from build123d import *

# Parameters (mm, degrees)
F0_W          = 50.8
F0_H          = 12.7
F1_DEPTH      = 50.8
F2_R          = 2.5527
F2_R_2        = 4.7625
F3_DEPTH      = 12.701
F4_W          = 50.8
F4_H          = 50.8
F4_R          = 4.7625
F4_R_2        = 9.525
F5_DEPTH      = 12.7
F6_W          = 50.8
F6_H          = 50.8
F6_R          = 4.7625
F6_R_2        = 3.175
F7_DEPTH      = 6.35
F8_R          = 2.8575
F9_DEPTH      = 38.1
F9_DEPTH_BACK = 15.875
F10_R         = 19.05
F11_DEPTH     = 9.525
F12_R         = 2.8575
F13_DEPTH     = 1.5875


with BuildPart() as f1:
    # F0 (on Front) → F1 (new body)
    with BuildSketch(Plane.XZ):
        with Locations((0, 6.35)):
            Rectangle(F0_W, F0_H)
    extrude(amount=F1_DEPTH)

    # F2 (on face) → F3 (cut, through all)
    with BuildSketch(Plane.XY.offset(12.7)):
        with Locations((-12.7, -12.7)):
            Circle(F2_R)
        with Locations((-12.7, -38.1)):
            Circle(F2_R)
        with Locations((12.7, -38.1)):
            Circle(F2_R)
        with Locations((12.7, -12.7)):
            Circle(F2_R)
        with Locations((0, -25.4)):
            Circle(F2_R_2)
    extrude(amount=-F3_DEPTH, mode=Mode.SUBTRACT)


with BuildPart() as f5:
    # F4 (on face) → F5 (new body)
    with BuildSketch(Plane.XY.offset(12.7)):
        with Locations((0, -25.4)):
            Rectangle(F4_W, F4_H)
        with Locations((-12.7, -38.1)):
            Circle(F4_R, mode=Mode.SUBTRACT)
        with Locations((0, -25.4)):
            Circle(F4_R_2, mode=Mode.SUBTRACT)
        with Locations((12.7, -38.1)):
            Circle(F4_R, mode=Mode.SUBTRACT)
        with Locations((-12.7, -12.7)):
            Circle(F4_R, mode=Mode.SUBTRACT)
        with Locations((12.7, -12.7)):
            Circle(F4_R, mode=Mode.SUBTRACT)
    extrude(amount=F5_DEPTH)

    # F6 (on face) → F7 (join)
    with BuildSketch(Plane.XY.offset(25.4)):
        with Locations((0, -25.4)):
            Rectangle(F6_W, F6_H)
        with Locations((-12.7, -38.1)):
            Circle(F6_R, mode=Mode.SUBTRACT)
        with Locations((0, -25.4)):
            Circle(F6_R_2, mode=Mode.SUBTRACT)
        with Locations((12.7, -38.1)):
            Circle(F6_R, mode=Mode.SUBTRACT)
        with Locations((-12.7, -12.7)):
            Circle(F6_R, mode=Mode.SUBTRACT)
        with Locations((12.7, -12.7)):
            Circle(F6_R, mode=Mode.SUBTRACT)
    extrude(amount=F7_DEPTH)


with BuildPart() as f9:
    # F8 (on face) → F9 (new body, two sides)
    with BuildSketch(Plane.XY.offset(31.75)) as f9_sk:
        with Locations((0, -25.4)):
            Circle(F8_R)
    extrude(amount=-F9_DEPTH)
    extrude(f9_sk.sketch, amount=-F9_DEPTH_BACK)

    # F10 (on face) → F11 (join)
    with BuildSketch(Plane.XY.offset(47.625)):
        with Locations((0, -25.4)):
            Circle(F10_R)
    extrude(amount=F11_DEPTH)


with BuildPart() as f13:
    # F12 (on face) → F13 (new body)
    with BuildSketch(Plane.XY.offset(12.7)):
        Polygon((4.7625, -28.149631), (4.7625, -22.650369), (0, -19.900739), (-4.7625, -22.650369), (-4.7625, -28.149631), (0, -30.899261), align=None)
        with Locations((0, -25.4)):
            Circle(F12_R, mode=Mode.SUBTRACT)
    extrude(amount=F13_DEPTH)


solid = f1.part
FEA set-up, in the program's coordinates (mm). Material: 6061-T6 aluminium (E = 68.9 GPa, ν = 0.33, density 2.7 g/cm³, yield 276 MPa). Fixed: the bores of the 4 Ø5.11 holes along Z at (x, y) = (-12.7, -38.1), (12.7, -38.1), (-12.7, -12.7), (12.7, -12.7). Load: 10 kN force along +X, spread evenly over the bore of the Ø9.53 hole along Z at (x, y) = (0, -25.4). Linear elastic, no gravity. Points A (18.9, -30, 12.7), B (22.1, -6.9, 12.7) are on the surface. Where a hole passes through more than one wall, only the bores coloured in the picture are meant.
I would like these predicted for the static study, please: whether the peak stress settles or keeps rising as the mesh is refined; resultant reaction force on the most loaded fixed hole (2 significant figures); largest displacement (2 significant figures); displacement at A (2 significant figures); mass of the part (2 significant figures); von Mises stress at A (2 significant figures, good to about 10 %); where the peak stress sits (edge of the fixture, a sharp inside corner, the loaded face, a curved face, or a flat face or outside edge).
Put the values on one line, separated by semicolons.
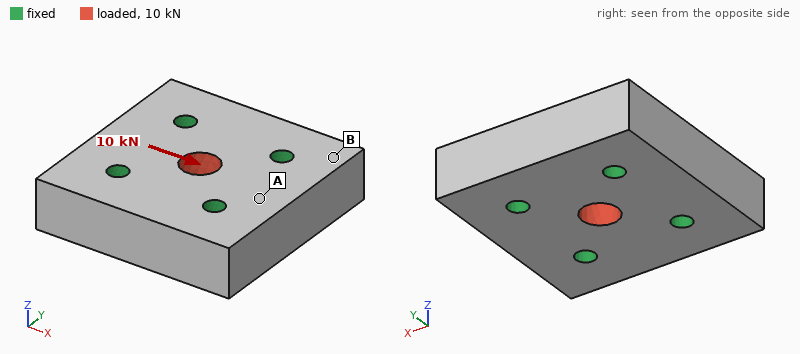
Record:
keeps rising; 2.7 kN; 5.2 µm; 1.9 µm; 83 g; 8.4 MPa; edge of the fixture
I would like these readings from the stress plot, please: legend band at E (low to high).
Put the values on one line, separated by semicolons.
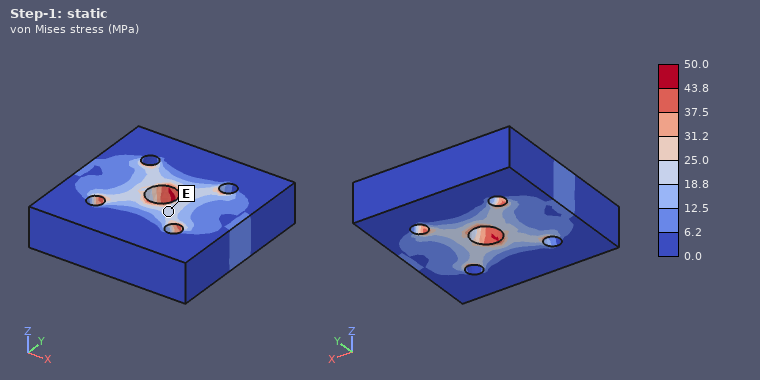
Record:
18.8 to 25.0 MPa
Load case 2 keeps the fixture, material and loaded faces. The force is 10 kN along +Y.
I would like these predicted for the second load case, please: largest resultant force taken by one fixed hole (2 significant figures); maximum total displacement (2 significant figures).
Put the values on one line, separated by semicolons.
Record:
2.7 kN; 5.1 µm
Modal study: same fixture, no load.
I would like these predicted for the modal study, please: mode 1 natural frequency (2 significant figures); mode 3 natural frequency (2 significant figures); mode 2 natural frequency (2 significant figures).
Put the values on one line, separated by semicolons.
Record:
35 kHz; 35 kHz; 35 kHz
